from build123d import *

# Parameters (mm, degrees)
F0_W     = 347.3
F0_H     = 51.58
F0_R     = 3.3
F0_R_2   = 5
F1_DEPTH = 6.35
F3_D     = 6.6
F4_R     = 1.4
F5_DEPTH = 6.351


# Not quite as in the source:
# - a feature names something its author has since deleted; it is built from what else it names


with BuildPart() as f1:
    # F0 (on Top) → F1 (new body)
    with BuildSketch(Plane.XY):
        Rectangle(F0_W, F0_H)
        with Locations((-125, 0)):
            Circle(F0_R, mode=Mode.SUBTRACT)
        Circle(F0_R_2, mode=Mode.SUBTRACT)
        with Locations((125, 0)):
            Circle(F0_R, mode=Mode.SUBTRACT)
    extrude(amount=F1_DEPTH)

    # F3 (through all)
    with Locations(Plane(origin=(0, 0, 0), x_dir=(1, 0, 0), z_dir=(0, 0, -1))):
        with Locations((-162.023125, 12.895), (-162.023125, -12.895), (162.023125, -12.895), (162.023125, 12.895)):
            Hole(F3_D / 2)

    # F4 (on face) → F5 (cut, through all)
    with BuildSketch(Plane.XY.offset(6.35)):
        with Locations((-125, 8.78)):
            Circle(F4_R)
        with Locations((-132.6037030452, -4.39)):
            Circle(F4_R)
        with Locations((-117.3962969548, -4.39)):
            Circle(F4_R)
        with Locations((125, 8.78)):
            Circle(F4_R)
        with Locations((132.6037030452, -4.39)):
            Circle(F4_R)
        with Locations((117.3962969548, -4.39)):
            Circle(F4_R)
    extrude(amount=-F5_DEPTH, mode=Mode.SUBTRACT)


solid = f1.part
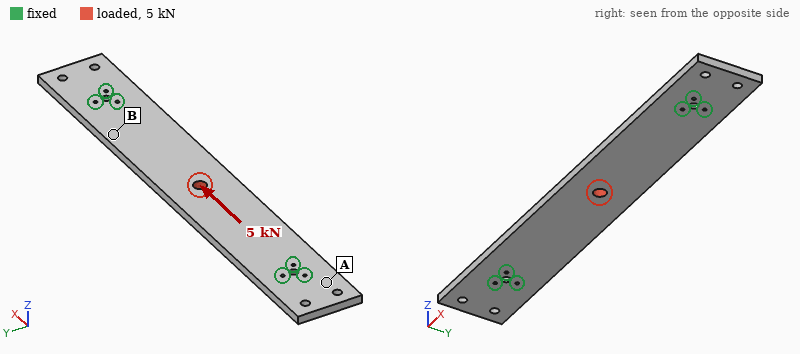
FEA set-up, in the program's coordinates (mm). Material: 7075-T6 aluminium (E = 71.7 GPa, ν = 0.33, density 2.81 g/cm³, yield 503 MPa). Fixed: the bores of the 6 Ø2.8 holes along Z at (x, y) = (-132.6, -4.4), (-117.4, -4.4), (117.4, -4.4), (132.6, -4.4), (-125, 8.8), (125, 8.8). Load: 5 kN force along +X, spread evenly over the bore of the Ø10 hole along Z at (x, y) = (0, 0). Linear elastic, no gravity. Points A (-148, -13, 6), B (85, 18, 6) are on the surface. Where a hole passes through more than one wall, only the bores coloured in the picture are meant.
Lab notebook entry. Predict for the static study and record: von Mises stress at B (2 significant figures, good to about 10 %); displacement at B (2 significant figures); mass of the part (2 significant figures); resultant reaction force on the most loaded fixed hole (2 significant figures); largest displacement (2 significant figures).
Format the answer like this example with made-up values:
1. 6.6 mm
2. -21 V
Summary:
1. 7.4 MPa
2. 5.1 µm
3. 310 g
4. 1.1 kN
5. 17 µm
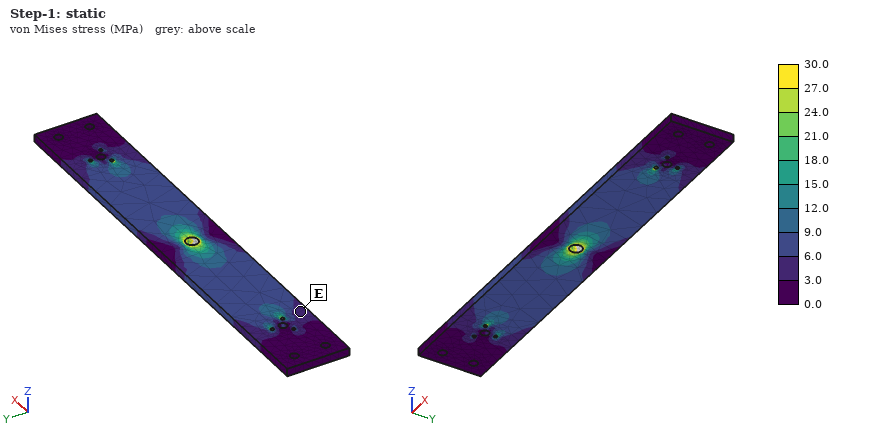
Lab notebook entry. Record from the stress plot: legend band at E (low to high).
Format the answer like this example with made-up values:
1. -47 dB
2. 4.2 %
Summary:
1. 3.0 to 6.0 MPa
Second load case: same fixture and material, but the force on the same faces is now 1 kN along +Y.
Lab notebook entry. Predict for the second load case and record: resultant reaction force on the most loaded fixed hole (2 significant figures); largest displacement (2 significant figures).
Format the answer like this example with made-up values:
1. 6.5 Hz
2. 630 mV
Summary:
1. 1.1 kN
2. 32 µm
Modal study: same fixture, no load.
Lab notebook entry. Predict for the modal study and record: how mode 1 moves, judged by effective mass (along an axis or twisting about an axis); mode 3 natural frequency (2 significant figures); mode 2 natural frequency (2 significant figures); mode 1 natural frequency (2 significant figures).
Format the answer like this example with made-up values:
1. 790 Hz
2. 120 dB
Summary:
1. along Z
2. 1600 Hz
3. 1500 Hz
4. 560 Hz
